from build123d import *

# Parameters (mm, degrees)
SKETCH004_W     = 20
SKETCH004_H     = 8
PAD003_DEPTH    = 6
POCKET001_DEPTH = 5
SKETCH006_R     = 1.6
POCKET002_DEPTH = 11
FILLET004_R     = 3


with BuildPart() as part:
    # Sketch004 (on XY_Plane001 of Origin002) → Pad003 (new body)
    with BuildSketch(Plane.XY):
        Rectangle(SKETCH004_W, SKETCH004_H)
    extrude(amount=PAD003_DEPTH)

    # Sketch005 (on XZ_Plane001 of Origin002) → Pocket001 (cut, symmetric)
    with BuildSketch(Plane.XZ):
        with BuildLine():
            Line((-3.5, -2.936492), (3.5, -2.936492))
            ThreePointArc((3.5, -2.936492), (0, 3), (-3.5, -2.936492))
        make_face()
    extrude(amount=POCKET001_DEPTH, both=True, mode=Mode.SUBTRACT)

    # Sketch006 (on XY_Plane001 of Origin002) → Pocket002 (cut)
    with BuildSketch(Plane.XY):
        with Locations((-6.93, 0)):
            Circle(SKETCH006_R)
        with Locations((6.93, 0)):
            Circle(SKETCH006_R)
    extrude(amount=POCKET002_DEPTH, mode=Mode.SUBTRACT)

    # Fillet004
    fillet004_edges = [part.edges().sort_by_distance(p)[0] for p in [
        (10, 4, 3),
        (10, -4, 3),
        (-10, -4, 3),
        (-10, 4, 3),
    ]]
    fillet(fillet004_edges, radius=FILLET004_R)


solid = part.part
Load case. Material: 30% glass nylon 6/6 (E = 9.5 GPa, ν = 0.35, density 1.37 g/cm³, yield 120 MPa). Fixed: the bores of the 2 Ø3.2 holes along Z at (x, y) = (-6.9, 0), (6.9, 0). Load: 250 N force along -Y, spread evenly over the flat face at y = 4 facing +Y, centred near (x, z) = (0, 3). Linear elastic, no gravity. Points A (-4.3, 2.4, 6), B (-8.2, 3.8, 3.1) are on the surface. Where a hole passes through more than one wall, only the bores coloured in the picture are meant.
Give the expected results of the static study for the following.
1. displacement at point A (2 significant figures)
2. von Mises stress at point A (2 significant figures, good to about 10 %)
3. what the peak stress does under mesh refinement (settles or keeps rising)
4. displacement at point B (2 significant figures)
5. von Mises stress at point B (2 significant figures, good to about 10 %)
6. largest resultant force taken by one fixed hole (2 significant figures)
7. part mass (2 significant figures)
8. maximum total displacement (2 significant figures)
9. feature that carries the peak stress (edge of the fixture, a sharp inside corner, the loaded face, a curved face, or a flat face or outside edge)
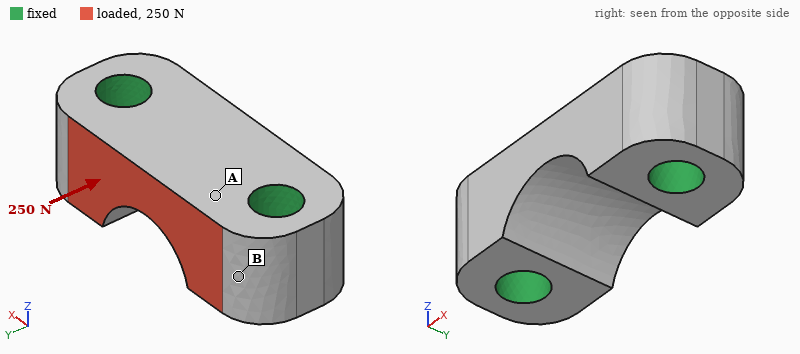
2.3 µm
5.1 MPa
keeps rising
0.81 µm
1.5 MPa
130 N
0.93 g
5.3 µm
edge of the fixture
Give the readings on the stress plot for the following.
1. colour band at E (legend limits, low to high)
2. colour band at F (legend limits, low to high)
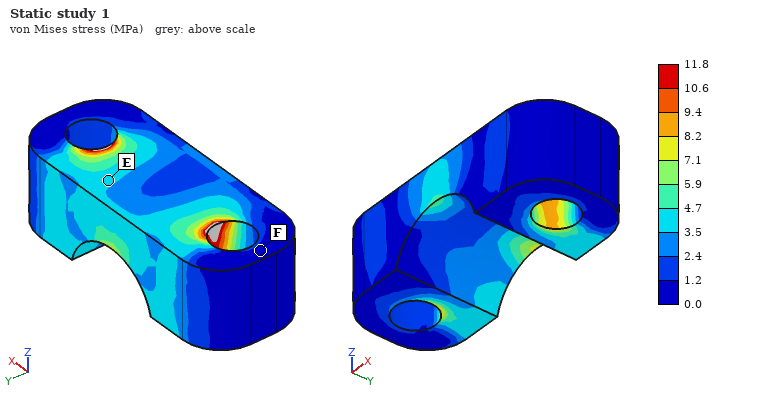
3.5 to 4.7 MPa
0.0 to 1.2 MPa
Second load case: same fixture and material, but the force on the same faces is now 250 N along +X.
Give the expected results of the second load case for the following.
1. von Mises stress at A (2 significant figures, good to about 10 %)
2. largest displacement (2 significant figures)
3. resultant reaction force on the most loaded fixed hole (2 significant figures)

6.0 MPa
4.7 µm
130 N
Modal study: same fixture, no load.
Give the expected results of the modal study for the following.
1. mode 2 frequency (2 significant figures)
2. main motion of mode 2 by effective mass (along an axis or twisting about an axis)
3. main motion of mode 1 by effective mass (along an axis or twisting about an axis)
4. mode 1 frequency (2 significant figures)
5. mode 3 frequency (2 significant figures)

59 kHz
along Z
along Y
54 kHz
71 kHz
